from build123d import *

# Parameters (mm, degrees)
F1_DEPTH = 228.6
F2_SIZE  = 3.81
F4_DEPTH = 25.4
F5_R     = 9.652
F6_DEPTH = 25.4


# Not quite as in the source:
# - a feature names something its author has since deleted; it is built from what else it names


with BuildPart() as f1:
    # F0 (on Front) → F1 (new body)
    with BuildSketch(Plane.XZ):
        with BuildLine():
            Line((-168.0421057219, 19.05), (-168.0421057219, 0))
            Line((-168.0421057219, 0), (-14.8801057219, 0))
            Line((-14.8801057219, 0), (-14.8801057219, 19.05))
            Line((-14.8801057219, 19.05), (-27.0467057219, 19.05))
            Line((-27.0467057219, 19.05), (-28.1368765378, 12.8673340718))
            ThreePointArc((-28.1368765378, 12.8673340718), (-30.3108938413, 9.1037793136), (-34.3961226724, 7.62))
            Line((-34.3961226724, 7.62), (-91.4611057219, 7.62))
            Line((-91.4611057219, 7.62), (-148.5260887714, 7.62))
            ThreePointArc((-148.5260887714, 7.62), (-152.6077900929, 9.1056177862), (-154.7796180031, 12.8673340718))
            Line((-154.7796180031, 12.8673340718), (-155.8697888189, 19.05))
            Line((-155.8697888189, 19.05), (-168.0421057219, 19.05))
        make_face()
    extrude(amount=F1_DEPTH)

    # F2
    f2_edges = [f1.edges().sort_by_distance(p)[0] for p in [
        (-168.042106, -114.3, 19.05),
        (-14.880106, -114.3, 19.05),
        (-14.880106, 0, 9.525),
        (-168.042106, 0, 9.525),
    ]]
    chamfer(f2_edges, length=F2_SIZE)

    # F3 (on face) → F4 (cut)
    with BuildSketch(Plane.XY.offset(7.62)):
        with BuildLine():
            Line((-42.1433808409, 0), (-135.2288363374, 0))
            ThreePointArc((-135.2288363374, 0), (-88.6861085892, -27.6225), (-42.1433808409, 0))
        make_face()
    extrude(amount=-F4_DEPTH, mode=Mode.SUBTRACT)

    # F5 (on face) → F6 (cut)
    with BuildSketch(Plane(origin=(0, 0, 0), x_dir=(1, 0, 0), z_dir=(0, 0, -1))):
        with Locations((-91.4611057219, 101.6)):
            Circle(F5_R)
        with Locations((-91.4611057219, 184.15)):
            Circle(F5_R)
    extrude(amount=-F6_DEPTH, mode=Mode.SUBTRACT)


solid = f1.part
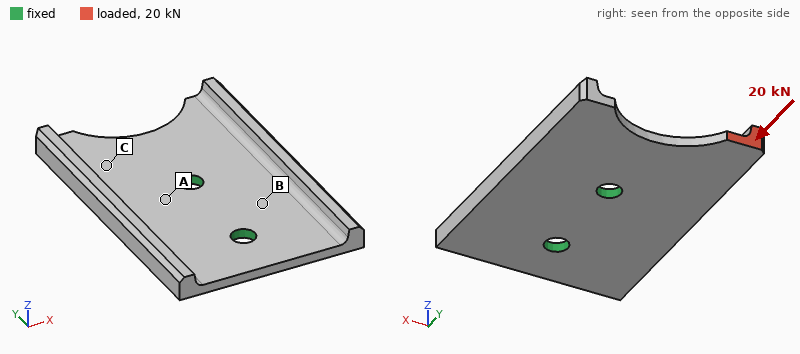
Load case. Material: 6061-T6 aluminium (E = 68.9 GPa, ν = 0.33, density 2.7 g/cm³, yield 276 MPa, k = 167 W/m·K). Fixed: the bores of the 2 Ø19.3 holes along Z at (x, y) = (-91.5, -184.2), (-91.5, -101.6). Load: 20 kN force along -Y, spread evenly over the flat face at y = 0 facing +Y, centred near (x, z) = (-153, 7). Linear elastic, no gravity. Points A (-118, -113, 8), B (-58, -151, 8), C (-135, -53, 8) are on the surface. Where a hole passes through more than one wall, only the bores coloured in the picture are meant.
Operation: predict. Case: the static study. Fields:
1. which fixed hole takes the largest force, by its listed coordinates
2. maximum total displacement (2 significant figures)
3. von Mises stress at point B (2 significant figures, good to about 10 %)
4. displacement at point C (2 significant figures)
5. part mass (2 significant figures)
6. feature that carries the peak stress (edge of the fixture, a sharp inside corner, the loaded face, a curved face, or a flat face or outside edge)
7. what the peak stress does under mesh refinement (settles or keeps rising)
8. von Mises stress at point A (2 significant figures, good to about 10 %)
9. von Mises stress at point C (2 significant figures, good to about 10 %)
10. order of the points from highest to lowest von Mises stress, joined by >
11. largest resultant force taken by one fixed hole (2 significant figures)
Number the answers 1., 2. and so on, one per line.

1. (-91.5, -101.6)
2. 0.31 mm
3. 13 MPa
4. 0.13 mm
5. 850 g
6. edge of the fixture
7. keeps rising
8. 53 MPa
9. 33 MPa
10. A > C > B
11. 18 kN
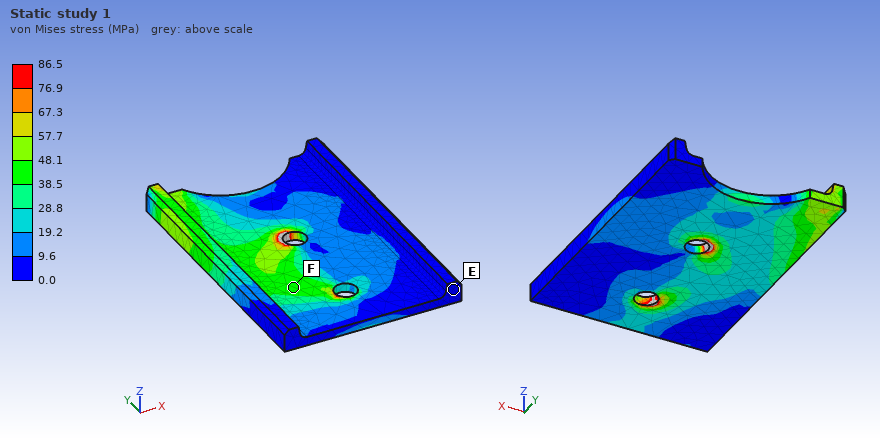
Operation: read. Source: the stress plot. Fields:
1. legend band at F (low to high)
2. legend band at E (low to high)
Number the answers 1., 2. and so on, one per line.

1. 38.5 to 48.1 MPa
2. 0.0 to 9.6 MPa
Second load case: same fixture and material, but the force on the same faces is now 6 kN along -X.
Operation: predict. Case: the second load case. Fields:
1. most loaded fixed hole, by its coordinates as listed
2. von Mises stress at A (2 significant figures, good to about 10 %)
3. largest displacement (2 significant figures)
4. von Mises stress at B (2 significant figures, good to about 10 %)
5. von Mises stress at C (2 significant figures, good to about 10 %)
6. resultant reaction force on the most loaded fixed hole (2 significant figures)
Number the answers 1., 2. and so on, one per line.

1. (-91.5, -101.6)
2. 17 MPa
3. 0.40 mm
4. 10.0 MPa
5. 21 MPa
6. 12 kN
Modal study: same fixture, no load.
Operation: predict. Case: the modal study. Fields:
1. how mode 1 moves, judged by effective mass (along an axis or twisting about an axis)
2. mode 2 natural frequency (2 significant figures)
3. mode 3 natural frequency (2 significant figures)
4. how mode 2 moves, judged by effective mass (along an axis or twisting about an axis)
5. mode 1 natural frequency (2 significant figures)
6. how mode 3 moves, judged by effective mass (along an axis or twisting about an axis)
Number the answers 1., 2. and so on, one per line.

1. twisting about Y
2. 690 Hz
3. 990 Hz
4. along Z
5. 620 Hz
6. along Z
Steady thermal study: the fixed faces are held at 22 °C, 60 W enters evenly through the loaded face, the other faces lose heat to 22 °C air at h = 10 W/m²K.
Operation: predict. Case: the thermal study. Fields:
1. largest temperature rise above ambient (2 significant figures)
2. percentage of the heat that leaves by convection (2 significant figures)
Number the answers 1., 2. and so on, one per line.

1. 66 K
2. 12 %
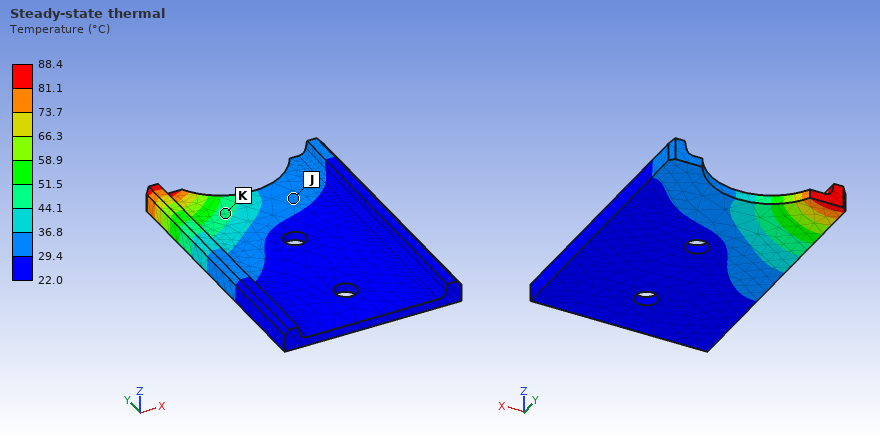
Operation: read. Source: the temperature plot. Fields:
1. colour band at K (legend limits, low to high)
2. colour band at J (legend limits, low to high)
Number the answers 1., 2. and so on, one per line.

1. 44.1 to 51.5 °C
2. 29.4 to 36.8 °C
